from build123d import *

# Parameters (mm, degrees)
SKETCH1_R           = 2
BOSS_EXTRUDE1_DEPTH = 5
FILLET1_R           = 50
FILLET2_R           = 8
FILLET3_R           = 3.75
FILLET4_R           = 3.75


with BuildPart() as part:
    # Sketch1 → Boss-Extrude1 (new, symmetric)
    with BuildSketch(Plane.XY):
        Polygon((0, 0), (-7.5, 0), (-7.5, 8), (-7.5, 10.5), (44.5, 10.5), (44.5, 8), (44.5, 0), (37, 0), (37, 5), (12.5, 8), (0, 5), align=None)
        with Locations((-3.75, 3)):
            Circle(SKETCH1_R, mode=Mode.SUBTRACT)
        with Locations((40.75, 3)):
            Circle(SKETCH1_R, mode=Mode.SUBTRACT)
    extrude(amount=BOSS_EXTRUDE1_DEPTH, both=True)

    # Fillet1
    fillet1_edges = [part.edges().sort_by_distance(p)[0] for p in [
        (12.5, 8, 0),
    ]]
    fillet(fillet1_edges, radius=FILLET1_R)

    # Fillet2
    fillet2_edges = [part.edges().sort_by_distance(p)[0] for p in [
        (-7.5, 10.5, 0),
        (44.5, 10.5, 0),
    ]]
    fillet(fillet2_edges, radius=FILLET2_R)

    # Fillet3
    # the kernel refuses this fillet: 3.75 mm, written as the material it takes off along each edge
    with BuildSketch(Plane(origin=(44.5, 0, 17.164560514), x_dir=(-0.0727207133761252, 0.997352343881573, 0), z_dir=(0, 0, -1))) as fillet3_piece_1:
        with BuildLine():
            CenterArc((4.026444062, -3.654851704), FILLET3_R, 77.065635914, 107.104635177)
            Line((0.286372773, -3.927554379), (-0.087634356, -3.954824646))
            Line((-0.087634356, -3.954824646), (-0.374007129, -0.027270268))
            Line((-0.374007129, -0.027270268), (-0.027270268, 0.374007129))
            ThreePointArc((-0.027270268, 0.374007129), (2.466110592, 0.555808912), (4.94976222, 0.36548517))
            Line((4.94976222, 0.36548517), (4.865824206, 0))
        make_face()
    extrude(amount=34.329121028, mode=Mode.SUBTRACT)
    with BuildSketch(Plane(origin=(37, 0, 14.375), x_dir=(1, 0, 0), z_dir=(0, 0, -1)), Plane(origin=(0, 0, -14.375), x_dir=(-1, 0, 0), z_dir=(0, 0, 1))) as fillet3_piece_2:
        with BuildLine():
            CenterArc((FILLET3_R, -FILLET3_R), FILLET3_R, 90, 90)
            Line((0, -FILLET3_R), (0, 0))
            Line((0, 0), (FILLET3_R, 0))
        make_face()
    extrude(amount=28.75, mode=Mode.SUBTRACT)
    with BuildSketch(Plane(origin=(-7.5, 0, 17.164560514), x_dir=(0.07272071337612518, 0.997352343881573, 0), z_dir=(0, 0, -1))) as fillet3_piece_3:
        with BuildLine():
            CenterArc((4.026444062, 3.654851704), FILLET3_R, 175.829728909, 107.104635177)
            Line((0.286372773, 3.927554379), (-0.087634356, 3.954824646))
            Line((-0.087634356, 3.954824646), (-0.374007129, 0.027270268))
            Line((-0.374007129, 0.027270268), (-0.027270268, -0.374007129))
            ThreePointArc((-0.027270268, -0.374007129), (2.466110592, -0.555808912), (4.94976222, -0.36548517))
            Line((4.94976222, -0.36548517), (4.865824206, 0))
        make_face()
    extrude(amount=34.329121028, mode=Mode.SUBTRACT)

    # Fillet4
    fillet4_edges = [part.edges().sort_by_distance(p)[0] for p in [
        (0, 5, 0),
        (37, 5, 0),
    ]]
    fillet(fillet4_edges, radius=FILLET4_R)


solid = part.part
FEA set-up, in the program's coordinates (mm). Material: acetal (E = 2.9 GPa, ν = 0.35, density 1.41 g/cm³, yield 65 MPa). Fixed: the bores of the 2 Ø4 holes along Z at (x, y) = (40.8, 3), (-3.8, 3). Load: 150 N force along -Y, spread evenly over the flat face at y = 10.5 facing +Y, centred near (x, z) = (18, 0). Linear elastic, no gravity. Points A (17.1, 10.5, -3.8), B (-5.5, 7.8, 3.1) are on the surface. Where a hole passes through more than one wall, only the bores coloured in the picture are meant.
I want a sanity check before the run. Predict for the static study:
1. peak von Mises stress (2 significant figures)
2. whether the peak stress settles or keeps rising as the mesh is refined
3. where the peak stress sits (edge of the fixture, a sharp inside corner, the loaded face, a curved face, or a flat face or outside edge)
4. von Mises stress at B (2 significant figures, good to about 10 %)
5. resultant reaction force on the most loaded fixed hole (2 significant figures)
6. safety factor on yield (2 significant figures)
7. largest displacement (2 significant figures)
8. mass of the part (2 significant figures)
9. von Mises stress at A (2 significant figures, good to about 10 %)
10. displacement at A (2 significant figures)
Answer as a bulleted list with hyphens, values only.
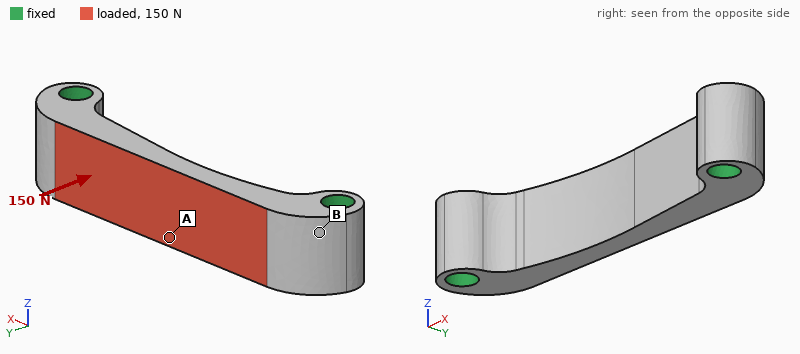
- 13 MPa
- settles
- a curved face
- 2.1 MPa
- 120 N
- 5.0
- 0.14 mm
- 3.5 g
- 10 MPa
- 0.14 mm
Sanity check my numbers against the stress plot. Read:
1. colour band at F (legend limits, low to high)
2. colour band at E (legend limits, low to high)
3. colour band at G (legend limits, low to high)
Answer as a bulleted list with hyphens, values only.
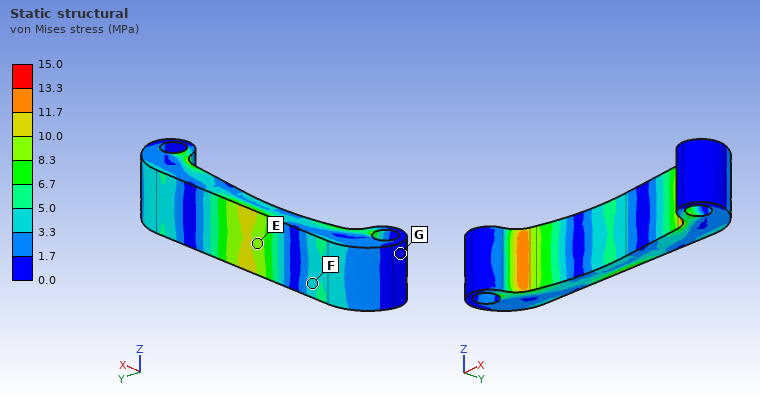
- 3.3 to 5.0 MPa
- 8.3 to 10.0 MPa
- 0.0 to 1.7 MPa
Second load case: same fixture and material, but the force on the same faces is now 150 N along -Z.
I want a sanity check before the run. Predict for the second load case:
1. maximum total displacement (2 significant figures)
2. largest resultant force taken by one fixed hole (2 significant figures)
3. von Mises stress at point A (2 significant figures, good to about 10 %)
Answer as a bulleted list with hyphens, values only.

- 88 µm
- 75 N
- 2.8 MPa
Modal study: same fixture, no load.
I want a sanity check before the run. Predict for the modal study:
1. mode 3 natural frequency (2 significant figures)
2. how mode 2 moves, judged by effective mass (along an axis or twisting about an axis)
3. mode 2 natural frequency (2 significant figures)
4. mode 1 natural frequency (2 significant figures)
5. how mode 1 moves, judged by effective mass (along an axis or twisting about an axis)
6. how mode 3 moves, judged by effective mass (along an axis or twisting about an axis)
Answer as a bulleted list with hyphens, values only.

- 8100 Hz
- along Z
- 6100 Hz
- 4400 Hz
- along Y
- along X
